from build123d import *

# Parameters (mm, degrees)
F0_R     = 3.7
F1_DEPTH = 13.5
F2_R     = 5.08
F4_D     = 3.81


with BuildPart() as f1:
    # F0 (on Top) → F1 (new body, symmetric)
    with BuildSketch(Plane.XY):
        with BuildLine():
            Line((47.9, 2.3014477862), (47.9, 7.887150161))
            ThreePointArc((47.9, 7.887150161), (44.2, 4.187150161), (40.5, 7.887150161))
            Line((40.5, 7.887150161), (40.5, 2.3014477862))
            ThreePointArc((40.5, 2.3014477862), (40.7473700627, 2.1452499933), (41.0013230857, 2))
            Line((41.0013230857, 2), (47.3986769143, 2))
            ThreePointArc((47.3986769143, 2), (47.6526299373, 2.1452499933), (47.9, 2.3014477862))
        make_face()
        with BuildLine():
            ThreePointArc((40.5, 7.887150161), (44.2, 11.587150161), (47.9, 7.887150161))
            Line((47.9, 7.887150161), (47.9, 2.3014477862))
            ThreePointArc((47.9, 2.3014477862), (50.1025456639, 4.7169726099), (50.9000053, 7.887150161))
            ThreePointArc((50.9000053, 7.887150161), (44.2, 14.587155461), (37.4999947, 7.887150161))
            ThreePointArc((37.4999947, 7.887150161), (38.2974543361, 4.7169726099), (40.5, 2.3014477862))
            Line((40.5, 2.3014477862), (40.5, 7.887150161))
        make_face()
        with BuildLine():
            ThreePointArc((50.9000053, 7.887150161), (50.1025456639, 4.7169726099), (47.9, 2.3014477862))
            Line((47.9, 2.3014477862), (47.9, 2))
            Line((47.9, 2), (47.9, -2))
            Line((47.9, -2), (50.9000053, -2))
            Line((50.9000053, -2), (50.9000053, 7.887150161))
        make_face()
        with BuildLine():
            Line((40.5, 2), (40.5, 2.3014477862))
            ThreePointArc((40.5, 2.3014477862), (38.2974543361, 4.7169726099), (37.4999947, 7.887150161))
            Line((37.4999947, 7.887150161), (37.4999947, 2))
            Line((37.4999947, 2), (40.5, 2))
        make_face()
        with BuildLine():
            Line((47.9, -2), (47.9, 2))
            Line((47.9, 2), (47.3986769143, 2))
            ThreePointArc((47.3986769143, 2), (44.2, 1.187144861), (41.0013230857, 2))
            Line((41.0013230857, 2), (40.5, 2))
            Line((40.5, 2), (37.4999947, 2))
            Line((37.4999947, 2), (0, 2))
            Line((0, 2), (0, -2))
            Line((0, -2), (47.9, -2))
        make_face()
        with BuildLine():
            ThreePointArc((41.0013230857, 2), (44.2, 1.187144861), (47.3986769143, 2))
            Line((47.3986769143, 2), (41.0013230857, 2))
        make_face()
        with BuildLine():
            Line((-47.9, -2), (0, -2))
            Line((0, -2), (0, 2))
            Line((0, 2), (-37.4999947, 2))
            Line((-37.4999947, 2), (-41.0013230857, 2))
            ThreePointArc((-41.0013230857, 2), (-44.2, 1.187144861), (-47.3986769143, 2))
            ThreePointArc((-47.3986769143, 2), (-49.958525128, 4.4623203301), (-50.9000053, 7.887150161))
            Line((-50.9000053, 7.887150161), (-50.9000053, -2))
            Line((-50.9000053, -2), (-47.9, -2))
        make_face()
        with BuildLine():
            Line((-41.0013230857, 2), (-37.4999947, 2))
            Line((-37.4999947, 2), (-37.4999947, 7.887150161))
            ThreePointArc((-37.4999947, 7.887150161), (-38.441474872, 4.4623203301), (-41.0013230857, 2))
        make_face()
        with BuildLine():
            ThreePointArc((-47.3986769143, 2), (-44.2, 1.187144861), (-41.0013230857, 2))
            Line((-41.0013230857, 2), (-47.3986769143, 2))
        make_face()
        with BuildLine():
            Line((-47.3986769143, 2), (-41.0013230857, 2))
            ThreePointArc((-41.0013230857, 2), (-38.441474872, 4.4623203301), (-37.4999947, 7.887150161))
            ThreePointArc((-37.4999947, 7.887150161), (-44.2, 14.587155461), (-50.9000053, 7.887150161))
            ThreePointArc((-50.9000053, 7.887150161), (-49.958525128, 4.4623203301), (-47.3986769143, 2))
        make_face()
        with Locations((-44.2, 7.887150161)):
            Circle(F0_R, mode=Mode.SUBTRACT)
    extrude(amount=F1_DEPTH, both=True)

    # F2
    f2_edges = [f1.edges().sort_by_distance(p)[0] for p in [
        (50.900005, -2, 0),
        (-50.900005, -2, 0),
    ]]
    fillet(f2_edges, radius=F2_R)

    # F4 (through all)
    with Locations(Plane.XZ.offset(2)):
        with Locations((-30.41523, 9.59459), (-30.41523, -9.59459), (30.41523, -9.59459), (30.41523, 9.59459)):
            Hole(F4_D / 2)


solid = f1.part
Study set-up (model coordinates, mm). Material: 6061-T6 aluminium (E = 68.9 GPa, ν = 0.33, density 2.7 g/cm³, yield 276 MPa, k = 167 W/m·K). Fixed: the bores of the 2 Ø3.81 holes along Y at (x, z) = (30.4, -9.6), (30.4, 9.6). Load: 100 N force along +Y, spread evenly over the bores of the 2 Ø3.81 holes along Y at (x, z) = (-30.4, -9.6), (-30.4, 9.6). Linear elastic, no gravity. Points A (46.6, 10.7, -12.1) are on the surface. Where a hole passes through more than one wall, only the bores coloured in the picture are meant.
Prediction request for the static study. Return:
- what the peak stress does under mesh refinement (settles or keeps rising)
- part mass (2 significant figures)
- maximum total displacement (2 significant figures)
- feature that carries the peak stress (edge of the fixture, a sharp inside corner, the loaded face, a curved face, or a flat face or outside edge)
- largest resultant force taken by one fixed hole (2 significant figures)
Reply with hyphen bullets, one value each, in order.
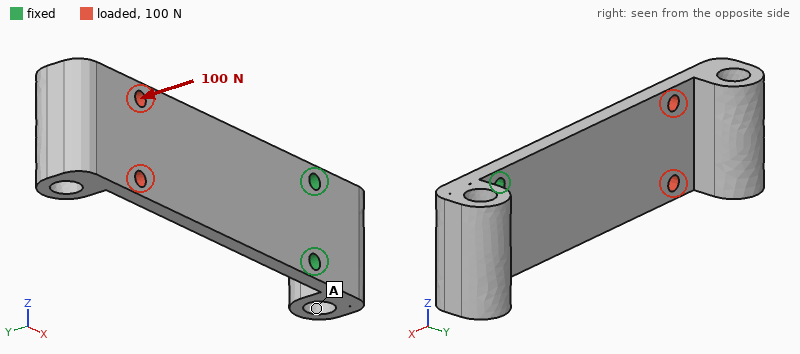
- keeps rising
- 44 g
- 1.1 mm
- edge of the fixture
- 50 N
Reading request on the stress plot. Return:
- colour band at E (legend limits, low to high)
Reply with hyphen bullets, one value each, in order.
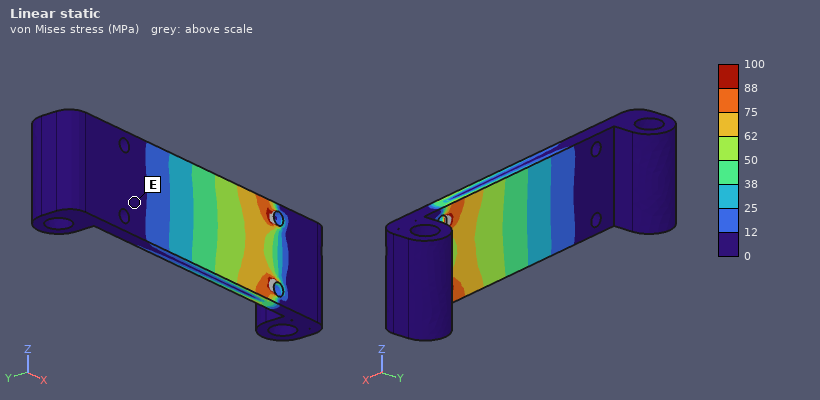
- 0 to 12 MPa
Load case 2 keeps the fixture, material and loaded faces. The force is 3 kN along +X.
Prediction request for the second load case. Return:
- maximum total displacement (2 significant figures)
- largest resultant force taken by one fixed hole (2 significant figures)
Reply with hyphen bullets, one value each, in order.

- 28 µm
- 1.5 kN
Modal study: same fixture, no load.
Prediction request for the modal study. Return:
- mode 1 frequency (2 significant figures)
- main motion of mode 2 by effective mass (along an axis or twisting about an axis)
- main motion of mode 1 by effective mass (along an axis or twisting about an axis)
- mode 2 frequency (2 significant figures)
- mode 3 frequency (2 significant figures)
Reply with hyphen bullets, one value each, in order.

- 350 Hz
- along Z
- along Y
- 1700 Hz
- 2500 Hz
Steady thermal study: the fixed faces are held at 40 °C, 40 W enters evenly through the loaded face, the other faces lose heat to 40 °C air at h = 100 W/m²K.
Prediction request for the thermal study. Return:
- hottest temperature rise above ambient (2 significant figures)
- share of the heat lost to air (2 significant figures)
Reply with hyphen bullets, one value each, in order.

- 66 K
- 63 %
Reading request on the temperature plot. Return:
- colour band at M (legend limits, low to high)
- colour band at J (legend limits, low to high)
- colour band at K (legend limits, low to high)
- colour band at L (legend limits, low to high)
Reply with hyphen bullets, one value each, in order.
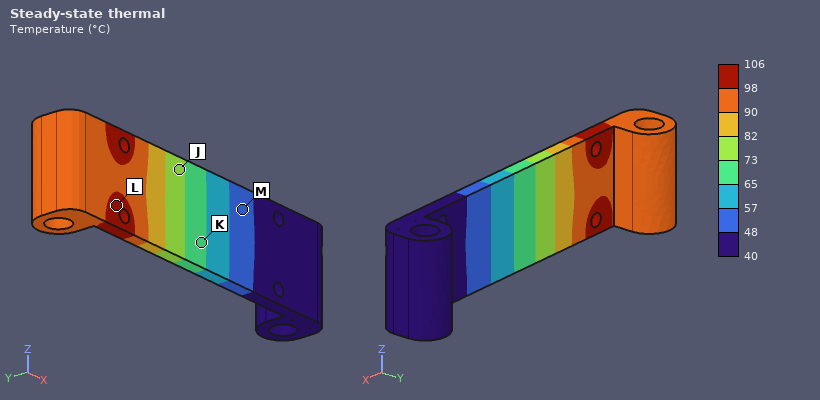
- 48 to 57 °C
- 73 to 82 °C
- 65 to 73 °C
- 98 to 106 °C
